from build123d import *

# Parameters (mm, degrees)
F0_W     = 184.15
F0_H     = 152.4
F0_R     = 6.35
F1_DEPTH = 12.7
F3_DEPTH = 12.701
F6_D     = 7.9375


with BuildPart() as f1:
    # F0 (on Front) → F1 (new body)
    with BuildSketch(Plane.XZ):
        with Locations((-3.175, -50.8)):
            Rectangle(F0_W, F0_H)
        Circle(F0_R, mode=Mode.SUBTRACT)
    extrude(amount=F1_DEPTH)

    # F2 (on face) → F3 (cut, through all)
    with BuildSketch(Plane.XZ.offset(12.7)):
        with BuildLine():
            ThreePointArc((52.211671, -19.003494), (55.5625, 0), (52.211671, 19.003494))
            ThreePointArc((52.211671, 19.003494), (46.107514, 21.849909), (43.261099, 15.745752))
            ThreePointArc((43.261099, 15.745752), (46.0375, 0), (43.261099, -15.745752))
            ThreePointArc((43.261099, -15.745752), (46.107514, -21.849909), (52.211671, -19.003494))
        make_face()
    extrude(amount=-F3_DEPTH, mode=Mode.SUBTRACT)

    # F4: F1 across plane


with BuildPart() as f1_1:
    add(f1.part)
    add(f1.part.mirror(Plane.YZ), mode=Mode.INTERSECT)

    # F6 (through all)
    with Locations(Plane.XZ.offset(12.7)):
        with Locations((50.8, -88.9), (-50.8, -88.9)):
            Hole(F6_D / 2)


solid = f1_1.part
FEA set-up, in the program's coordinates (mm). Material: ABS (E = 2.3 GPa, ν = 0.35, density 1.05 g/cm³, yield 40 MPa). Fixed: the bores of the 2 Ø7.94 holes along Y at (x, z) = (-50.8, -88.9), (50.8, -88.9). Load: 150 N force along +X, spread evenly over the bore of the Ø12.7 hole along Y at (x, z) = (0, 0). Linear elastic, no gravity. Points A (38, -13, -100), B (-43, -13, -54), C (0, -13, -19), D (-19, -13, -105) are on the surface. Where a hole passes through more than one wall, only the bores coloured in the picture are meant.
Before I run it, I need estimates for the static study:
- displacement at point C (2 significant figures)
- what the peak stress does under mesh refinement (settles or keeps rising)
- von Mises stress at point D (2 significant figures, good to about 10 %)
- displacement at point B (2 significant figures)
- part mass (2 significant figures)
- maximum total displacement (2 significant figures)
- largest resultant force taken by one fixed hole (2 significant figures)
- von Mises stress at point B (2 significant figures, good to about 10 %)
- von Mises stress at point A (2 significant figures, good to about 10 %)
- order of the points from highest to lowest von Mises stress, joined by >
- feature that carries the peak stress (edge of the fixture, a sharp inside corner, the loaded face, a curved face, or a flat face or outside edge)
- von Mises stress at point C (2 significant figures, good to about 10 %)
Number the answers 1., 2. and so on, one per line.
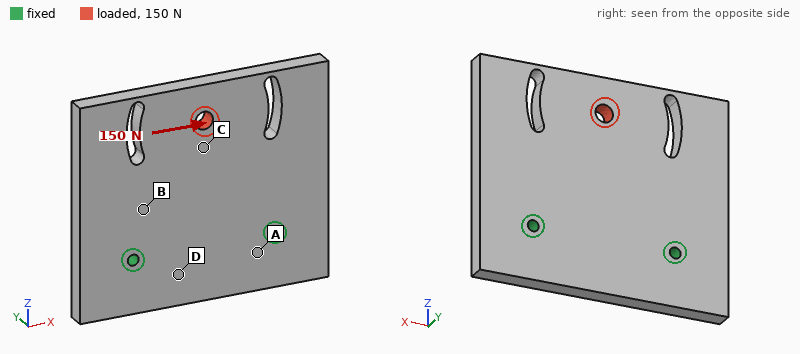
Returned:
1. 13 µm
2. keeps rising
3. 0.051 MPa
4. 6.6 µm
5. 350 g
6. 21 µm
7. 150 N
8. 0.20 MPa
9. 0.090 MPa
10. C > B > A > D
11. edge of the fixture
12. 0.26 MPa
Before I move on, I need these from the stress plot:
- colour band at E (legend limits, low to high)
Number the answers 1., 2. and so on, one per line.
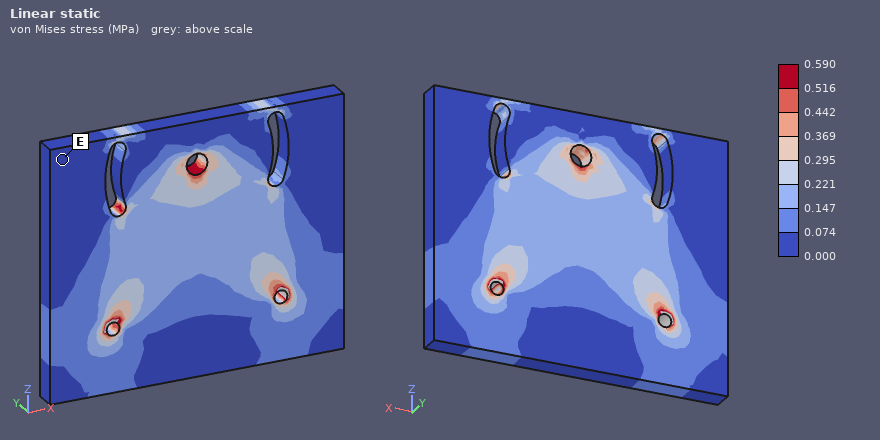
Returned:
1. 0.000 to 0.074 MPa
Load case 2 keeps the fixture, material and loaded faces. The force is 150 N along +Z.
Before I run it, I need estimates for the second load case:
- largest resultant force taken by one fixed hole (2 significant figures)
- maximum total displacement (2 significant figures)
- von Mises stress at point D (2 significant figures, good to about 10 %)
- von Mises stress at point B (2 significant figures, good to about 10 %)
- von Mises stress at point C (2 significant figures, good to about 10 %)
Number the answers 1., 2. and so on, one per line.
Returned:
1. 78 N
2. 9.1 µm
3. 0.049 MPa
4. 0.12 MPa
5. 0.22 MPa
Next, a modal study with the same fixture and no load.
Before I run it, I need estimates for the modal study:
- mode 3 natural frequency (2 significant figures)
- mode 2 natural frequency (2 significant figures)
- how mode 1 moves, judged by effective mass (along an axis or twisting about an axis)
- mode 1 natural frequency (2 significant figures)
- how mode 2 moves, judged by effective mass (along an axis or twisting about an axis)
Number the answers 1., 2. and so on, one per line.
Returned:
1. 720 Hz
2. 370 Hz
3. along Y
4. 210 Hz
5. twisting about Z
